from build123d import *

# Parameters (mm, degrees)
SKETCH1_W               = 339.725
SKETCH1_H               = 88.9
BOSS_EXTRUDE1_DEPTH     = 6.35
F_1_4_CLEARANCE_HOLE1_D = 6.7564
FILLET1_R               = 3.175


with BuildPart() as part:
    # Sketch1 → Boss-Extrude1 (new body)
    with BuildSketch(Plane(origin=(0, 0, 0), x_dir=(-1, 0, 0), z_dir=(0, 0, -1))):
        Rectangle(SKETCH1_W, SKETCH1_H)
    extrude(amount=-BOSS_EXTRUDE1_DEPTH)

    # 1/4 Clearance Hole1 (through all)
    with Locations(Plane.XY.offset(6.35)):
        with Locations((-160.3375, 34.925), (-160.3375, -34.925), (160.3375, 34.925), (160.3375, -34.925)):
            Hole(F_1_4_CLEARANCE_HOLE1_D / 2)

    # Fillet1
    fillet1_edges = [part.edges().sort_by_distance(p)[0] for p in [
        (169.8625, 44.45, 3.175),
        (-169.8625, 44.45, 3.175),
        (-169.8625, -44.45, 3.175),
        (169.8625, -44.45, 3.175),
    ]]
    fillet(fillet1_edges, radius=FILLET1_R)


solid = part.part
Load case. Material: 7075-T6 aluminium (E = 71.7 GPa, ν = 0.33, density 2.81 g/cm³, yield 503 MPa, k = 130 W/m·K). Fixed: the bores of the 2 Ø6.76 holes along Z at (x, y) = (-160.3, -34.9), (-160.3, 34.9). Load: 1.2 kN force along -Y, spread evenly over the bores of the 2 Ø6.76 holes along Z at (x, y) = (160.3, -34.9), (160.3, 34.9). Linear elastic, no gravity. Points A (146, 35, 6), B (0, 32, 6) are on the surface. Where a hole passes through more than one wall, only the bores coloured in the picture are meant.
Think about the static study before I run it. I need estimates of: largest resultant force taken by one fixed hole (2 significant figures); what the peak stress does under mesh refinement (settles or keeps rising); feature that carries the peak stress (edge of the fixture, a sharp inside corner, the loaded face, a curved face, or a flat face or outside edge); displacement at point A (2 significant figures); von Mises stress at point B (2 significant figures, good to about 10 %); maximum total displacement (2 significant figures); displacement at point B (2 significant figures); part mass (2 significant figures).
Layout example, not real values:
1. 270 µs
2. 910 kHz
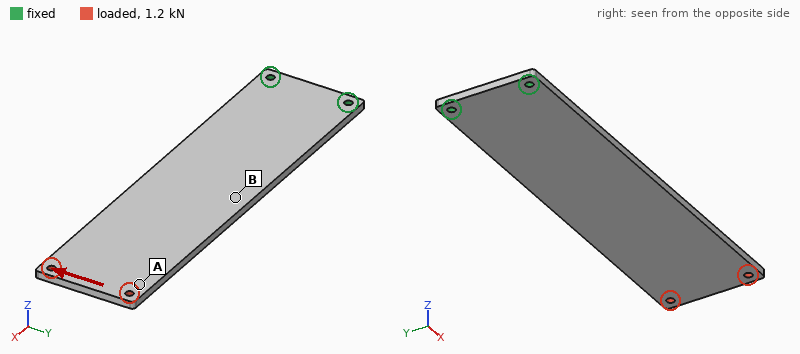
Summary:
1. 5.4 kN
2. keeps rising
3. edge of the fixture
4. 0.51 mm
5. 17 MPa
6. 0.57 mm
7. 0.19 mm
8. 540 g
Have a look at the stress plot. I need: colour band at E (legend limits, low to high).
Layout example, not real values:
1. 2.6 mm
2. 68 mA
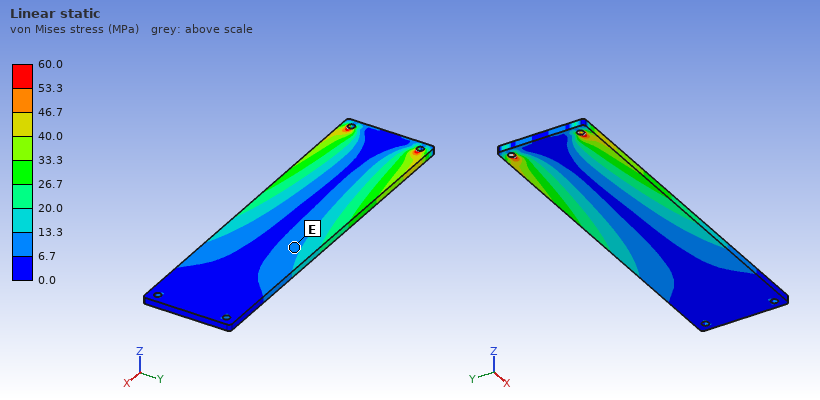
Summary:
1. 6.7 to 13.3 MPa
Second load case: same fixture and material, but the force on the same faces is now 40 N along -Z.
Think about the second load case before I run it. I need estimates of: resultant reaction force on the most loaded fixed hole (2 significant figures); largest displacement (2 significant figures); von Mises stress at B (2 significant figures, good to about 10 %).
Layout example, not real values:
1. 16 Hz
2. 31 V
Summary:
1. 20 N
2. 3.5 mm
3. 11 MPa
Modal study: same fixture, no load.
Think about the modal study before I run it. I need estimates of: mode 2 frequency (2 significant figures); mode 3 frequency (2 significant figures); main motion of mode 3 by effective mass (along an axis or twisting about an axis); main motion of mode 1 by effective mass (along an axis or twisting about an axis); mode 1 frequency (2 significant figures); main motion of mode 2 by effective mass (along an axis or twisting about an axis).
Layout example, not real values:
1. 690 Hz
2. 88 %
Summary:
1. 290 Hz
2. 350 Hz
3. twisting about X
4. along Z
5. 46 Hz
6. along Z
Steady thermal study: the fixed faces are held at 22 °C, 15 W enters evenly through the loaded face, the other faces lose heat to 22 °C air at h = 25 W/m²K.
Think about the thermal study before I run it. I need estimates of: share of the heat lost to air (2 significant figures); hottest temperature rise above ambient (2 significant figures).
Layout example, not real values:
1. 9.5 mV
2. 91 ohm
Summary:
1. 87 %
2. 26 K
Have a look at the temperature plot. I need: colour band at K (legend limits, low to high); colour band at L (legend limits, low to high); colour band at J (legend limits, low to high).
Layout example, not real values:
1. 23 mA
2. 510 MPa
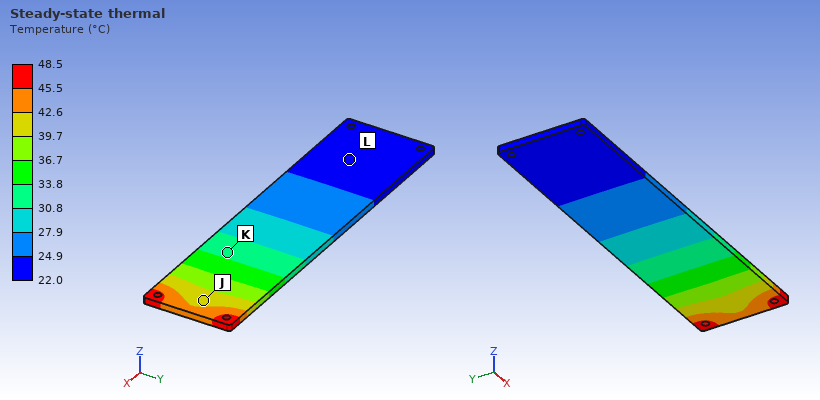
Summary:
1. 30.8 to 33.8 °C
2. 22.0 to 24.9 °C
3. 39.7 to 42.6 °C
